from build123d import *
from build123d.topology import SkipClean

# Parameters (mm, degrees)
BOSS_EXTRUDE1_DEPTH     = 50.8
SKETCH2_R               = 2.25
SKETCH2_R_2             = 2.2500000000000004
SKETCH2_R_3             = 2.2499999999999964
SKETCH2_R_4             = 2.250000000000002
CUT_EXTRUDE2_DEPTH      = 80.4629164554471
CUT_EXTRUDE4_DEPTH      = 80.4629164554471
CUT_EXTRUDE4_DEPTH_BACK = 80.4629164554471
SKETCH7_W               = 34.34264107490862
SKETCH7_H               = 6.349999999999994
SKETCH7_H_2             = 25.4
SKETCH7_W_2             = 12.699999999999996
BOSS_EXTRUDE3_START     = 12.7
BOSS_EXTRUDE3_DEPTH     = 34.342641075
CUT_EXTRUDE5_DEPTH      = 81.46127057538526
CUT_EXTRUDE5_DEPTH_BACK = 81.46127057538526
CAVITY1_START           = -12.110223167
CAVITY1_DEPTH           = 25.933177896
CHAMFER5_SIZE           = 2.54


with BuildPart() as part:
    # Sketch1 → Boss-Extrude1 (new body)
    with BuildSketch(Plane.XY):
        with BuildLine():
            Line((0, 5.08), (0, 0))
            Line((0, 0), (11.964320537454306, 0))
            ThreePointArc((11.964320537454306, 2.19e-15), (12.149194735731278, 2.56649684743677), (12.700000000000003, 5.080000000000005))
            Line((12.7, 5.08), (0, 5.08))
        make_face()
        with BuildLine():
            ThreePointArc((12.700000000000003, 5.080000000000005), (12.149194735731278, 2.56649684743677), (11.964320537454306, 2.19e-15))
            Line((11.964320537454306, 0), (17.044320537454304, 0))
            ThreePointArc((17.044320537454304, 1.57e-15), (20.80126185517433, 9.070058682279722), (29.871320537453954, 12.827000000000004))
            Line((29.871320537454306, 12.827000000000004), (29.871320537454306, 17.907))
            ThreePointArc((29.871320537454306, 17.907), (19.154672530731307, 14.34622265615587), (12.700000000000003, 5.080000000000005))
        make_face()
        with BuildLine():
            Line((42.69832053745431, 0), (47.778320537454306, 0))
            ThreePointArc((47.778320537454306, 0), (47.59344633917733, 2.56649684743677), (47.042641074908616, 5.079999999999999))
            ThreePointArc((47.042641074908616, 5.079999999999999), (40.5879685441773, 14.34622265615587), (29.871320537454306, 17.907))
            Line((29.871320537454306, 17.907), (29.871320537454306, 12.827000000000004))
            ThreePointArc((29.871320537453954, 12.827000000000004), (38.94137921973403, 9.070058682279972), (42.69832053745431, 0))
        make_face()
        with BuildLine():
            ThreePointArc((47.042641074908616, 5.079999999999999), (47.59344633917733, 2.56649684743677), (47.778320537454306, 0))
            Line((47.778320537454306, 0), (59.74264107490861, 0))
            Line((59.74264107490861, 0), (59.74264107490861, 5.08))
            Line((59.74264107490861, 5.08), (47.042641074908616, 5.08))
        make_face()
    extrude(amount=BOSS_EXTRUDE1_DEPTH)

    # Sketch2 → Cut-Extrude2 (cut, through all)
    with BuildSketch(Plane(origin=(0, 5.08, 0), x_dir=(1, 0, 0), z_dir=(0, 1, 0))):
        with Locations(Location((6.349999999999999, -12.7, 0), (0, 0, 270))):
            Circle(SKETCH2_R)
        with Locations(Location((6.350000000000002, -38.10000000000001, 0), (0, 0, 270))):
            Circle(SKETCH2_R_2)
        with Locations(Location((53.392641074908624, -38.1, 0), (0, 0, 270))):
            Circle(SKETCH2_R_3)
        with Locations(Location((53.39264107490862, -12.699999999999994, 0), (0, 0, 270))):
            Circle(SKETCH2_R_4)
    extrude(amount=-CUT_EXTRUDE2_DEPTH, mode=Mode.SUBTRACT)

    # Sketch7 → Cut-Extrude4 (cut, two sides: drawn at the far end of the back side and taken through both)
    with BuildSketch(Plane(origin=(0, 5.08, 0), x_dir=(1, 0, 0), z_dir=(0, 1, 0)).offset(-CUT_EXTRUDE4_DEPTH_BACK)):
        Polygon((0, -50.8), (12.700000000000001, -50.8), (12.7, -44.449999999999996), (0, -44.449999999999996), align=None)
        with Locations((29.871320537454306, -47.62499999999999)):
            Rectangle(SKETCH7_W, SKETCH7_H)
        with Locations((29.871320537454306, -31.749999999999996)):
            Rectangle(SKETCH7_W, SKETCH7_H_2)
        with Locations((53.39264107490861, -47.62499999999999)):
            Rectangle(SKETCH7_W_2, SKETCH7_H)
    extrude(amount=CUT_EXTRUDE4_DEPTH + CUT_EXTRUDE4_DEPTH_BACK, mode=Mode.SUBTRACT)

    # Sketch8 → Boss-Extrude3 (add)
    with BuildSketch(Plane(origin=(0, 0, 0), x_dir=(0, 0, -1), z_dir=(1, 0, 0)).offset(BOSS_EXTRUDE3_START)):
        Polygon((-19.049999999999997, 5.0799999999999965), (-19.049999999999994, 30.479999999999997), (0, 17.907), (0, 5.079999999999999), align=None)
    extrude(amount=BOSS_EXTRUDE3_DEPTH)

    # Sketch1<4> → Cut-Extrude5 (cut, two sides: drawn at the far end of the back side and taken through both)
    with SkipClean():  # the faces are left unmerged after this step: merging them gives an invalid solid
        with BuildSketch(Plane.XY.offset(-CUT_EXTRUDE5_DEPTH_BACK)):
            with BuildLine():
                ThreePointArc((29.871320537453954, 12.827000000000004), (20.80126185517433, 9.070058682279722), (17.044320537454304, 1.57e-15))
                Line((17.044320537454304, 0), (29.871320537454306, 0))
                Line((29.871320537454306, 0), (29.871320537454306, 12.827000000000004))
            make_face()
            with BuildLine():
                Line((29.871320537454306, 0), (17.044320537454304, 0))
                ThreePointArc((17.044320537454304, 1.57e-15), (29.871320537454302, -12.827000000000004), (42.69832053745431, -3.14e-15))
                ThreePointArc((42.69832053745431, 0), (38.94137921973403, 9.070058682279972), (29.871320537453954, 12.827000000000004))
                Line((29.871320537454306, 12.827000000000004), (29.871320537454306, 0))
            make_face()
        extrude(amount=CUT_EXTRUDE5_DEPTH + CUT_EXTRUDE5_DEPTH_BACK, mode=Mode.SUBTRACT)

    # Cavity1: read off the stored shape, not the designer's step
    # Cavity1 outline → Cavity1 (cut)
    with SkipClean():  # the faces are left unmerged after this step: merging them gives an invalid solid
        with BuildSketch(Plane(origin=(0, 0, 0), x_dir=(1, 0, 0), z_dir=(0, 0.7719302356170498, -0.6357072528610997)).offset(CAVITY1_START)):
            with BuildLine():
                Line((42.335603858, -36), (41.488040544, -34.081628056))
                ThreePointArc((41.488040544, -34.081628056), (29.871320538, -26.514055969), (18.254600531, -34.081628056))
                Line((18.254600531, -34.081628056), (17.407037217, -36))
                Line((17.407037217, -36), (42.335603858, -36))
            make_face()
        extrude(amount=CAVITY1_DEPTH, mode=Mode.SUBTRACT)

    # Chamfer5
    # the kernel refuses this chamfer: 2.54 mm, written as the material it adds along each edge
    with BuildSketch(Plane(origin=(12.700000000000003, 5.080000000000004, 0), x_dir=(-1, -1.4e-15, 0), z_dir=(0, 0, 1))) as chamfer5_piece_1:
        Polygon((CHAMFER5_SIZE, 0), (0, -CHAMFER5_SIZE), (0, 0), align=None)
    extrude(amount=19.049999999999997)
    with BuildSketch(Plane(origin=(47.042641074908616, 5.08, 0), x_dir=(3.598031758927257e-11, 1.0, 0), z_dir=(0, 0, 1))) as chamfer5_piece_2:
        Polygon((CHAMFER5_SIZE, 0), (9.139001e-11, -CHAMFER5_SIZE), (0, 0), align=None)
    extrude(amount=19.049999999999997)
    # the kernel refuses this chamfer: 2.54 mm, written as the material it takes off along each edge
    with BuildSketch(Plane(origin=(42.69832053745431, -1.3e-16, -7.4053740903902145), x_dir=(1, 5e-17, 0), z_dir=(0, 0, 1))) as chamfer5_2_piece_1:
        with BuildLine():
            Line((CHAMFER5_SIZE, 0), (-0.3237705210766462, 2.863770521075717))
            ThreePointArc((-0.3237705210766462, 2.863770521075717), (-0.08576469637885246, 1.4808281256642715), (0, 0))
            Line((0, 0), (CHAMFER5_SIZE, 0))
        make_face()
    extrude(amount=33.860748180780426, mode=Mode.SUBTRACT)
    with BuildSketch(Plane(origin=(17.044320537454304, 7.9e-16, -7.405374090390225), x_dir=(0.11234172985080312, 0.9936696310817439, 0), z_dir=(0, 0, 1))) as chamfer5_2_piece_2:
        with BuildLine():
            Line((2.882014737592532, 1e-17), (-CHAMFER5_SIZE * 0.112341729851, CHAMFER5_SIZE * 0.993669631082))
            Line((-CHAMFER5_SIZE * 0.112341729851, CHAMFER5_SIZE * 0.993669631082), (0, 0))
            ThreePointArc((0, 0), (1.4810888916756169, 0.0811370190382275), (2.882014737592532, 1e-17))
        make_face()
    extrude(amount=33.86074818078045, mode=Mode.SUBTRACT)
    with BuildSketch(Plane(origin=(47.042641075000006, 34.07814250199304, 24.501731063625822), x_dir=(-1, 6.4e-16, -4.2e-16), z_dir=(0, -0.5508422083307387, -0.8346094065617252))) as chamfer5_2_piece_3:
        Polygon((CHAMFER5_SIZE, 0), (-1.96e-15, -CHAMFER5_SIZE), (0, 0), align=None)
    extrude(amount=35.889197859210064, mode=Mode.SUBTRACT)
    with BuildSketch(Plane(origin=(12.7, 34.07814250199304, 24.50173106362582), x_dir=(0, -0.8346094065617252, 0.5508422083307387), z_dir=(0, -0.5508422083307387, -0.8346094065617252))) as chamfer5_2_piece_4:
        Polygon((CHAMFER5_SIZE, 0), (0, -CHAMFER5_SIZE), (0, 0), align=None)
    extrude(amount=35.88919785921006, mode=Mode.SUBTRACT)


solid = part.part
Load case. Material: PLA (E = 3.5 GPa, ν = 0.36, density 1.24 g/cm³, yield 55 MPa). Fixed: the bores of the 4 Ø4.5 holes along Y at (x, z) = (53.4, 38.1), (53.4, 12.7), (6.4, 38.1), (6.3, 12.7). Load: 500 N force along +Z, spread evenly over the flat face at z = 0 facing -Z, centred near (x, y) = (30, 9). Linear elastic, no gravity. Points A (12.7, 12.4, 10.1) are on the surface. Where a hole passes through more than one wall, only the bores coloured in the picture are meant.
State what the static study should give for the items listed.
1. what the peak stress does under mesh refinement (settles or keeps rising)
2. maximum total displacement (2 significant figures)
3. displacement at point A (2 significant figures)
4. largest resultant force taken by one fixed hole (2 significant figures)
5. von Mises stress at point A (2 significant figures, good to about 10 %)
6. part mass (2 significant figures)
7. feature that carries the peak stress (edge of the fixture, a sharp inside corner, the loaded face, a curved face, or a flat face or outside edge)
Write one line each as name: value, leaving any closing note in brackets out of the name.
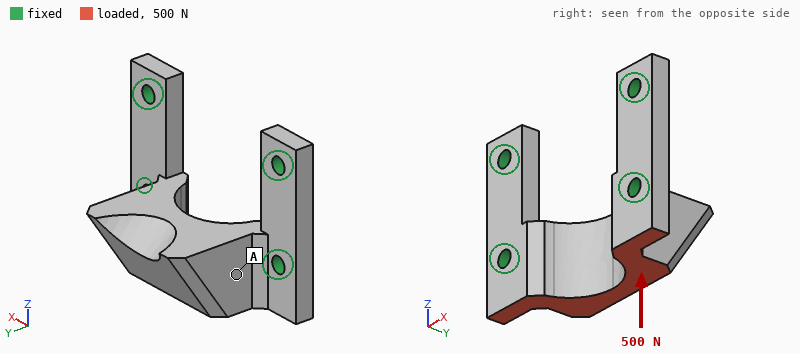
what the peak stress does under mesh refinement: keeps rising
maximum total displacement: 0.28 mm
displacement at point A: 0.11 mm
largest resultant force taken by one fixed hole: 210 N
von Mises stress at point A: 3.1 MPa
part mass: 19 g
feature that carries the peak stress: edge of the fixture
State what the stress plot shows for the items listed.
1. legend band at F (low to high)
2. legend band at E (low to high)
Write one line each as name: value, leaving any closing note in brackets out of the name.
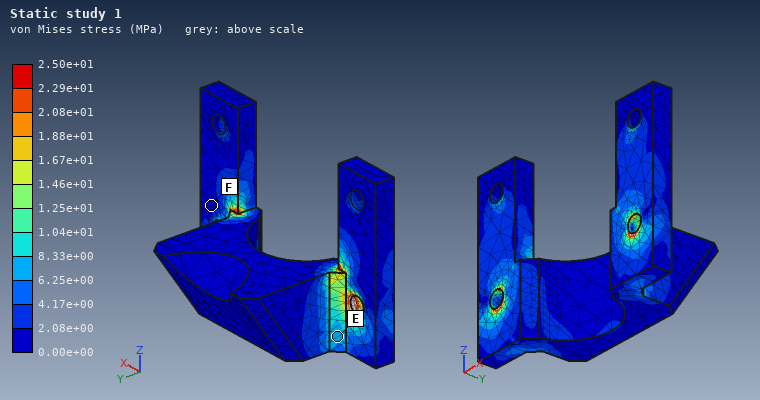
legend band at F: 0.00e+00 to 2.08e+00 MPa
legend band at E: 6.25e+00 to 8.33e+00 MPa
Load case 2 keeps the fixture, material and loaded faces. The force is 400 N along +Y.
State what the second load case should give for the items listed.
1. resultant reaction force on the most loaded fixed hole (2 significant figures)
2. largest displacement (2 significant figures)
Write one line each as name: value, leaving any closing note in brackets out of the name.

resultant reaction force on the most loaded fixed hole: 250 N
largest displacement: 0.35 mm
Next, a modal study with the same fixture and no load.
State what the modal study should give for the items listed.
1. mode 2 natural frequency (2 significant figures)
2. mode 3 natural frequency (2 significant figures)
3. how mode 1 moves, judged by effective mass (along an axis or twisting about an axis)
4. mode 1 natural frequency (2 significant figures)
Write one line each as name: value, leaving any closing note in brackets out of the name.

mode 2 natural frequency: 5000 Hz
mode 3 natural frequency: 5100 Hz
how mode 1 moves, judged by effective mass: along Z
mode 1 natural frequency: 1700 Hz
